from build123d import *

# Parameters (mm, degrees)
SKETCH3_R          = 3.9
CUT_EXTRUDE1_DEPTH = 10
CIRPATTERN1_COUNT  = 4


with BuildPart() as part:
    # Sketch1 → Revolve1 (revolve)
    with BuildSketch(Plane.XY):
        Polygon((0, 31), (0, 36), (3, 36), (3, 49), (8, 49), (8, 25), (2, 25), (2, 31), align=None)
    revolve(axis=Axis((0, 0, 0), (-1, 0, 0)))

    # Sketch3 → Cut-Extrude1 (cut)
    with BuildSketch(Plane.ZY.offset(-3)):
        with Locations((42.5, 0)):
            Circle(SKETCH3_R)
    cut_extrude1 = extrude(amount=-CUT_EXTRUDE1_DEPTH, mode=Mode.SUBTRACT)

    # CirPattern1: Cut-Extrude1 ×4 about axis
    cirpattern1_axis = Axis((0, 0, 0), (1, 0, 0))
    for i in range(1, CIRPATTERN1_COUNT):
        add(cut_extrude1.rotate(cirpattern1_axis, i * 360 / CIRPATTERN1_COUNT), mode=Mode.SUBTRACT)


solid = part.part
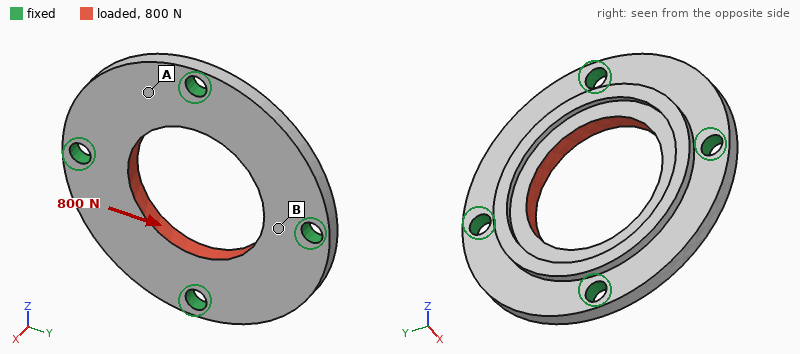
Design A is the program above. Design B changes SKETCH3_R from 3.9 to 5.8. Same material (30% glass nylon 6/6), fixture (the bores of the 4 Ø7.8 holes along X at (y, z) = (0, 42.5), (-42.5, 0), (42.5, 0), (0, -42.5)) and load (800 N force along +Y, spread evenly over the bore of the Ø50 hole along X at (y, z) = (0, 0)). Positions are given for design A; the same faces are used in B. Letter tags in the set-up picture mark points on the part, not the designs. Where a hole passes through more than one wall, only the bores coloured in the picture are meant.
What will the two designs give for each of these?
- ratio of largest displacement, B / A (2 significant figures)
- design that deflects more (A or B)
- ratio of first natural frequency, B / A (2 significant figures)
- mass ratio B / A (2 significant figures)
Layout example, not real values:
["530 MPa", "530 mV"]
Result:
["0.83", "A", "1.2", "0.96"]
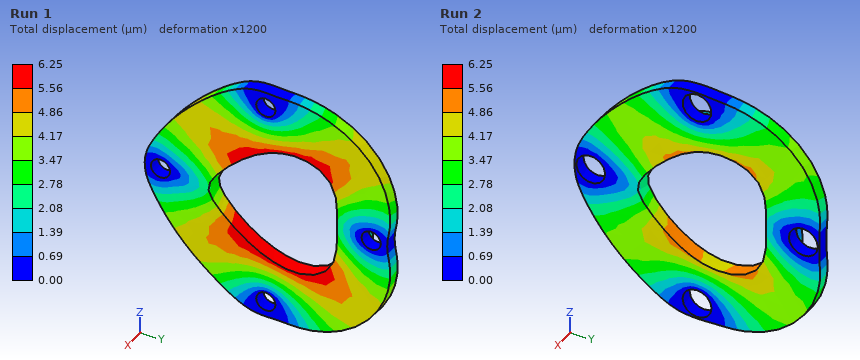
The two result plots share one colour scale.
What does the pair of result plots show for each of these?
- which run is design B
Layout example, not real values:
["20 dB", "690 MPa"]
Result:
["Run 2"]
